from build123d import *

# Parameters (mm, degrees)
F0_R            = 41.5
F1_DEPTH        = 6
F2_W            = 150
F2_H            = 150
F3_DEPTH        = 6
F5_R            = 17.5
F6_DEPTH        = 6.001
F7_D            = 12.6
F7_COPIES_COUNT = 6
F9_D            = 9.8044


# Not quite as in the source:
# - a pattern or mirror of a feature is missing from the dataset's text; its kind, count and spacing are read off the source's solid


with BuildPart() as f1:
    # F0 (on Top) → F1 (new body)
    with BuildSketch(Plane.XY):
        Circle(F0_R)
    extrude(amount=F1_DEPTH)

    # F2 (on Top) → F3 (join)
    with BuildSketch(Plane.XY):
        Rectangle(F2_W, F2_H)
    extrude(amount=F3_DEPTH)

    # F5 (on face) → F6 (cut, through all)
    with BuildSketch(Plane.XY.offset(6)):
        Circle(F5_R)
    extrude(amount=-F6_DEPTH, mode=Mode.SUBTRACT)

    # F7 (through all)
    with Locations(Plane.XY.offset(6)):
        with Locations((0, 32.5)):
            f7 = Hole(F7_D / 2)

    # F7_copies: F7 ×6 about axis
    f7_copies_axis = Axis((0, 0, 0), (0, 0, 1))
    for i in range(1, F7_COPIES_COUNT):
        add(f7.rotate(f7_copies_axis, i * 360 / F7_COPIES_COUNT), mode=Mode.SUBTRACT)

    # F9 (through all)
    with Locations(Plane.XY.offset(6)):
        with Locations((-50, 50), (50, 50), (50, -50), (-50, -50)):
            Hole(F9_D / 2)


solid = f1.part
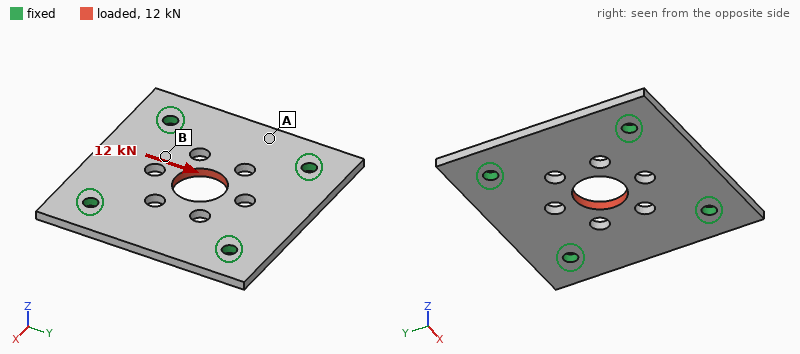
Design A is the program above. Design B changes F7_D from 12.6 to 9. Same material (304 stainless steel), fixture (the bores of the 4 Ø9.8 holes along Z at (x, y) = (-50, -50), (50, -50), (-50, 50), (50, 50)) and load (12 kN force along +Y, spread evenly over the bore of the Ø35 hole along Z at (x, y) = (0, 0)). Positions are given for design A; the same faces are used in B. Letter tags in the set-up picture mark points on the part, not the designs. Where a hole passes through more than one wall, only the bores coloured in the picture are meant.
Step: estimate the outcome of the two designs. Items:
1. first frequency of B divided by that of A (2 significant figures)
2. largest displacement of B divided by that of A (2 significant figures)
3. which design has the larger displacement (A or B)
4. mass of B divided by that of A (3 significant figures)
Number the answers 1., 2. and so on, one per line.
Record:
1. 0.99
2. 0.90
3. A
4. 1.02
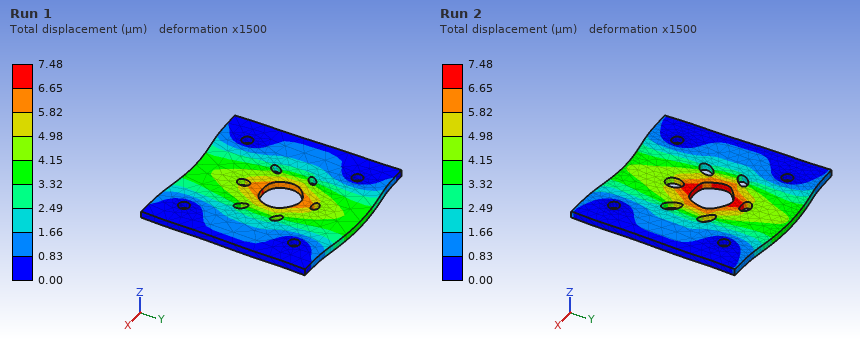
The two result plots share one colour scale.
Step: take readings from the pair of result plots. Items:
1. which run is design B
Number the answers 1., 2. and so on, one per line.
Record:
1. Run 1
